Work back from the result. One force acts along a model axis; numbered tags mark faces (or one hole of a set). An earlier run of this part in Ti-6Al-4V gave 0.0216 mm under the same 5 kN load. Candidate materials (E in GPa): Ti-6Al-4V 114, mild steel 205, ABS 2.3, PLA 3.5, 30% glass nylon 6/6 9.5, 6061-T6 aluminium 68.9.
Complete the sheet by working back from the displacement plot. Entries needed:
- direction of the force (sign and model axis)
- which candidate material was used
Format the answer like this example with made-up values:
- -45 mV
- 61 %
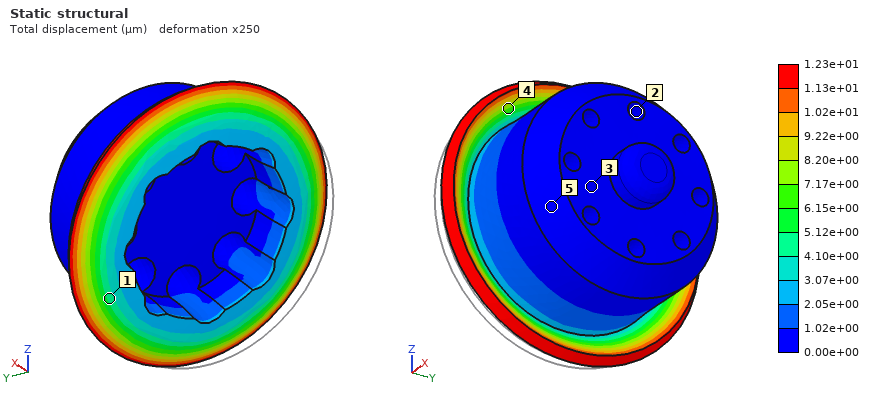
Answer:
- +X
- mild steel
